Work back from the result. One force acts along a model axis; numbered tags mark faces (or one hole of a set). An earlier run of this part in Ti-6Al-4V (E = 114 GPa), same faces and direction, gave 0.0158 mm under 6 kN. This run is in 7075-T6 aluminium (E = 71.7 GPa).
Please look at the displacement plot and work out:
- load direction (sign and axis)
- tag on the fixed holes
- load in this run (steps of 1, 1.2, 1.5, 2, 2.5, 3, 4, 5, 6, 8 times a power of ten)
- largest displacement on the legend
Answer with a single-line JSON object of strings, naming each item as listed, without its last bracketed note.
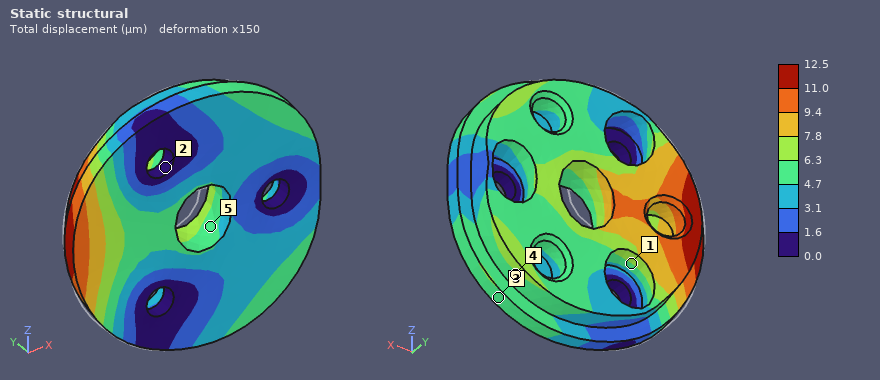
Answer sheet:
{"load direction": "+X", "tag on the fixed holes": "2", "load in this run": "3 kN", "largest displacement on the legend": "12.5 µm"}
